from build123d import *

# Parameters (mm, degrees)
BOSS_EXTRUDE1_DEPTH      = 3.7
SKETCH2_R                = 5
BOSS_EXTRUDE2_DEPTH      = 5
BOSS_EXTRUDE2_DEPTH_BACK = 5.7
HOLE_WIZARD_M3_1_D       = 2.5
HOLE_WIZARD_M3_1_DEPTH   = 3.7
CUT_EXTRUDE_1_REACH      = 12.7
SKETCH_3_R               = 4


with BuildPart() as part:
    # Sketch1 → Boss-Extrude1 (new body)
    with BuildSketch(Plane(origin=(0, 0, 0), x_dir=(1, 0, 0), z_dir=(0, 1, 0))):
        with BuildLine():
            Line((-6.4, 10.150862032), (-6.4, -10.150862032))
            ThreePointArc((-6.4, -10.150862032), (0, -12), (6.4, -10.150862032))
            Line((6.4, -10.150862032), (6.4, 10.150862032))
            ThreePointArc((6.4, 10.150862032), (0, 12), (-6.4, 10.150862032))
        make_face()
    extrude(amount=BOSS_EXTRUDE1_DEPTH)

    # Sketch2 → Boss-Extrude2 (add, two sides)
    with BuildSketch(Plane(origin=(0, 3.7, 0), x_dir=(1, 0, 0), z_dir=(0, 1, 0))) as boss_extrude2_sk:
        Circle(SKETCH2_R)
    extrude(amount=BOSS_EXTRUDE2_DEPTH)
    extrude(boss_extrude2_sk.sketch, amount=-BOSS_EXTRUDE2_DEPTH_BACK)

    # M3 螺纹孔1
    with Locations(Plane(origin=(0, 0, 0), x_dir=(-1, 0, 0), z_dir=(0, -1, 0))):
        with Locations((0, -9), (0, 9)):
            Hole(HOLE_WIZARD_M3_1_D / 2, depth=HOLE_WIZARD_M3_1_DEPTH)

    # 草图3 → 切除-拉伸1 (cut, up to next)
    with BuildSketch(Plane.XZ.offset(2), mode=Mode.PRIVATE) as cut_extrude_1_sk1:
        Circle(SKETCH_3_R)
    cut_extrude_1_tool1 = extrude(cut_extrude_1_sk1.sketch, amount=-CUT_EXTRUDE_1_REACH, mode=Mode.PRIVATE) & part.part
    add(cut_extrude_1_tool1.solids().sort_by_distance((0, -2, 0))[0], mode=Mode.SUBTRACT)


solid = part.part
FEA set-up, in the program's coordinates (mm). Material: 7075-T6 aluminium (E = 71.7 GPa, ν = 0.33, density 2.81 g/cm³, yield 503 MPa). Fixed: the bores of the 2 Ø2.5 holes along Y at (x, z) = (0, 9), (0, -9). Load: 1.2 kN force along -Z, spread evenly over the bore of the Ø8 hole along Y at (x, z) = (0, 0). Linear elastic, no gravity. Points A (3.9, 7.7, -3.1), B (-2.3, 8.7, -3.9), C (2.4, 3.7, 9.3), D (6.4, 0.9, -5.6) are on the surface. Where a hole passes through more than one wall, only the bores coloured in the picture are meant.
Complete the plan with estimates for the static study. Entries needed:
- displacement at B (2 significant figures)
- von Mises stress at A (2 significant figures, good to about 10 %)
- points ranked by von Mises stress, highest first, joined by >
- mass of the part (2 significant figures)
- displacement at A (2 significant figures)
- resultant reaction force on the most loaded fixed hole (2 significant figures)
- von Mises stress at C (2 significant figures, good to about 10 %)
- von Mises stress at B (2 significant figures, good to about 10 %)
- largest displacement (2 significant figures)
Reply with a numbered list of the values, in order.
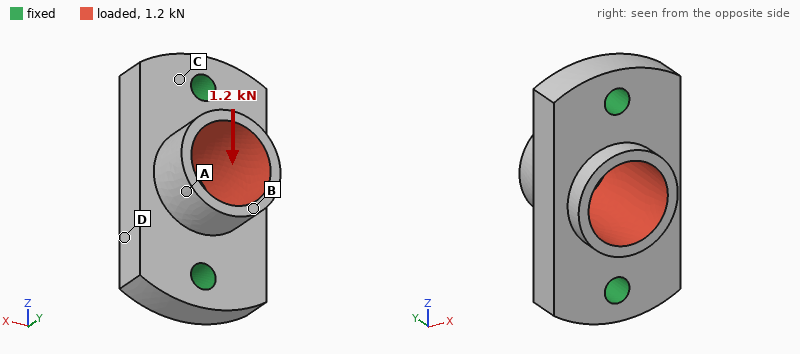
1. 8.9 µm
2. 17 MPa
3. B > A > C > D
4. 3.0 g
5. 7.5 µm
6. 610 N
7. 11 MPa
8. 26 MPa
9. 9.2 µm
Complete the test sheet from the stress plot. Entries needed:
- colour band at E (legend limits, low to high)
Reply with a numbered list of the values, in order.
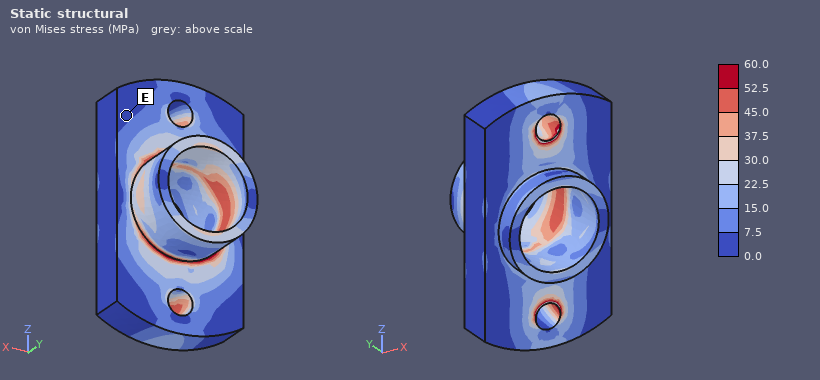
1. 0.0 to 7.5 MPa
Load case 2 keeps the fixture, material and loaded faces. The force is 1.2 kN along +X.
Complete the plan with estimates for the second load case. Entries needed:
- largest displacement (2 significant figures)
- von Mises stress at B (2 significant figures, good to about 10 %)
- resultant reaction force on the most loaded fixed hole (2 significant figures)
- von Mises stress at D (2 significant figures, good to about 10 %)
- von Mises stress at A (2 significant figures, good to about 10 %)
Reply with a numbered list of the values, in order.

1. 20 µm
2. 14 MPa
3. 600 N
4. 16 MPa
5. 15 MPa
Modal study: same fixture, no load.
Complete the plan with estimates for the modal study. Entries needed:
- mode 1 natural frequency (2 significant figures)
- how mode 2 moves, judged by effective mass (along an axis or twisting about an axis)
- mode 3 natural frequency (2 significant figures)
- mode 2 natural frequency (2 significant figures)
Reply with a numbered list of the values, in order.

1. 32 kHz
2. along Y
3. 54 kHz
4. 39 kHz
